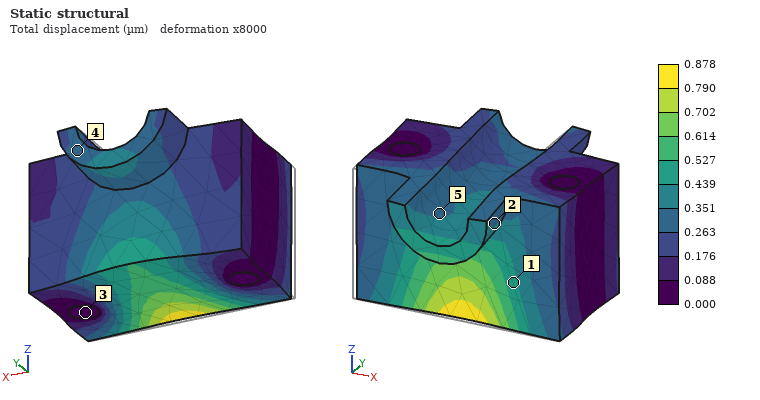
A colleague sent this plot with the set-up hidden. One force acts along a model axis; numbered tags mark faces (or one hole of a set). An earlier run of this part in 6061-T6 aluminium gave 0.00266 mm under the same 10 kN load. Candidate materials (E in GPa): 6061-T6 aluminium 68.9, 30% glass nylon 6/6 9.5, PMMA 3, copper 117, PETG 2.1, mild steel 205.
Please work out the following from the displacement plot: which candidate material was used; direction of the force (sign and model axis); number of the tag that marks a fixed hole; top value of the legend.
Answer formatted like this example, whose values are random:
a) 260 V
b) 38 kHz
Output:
a) mild steel
b) +Y
c) 3
d) 0.878 µm
